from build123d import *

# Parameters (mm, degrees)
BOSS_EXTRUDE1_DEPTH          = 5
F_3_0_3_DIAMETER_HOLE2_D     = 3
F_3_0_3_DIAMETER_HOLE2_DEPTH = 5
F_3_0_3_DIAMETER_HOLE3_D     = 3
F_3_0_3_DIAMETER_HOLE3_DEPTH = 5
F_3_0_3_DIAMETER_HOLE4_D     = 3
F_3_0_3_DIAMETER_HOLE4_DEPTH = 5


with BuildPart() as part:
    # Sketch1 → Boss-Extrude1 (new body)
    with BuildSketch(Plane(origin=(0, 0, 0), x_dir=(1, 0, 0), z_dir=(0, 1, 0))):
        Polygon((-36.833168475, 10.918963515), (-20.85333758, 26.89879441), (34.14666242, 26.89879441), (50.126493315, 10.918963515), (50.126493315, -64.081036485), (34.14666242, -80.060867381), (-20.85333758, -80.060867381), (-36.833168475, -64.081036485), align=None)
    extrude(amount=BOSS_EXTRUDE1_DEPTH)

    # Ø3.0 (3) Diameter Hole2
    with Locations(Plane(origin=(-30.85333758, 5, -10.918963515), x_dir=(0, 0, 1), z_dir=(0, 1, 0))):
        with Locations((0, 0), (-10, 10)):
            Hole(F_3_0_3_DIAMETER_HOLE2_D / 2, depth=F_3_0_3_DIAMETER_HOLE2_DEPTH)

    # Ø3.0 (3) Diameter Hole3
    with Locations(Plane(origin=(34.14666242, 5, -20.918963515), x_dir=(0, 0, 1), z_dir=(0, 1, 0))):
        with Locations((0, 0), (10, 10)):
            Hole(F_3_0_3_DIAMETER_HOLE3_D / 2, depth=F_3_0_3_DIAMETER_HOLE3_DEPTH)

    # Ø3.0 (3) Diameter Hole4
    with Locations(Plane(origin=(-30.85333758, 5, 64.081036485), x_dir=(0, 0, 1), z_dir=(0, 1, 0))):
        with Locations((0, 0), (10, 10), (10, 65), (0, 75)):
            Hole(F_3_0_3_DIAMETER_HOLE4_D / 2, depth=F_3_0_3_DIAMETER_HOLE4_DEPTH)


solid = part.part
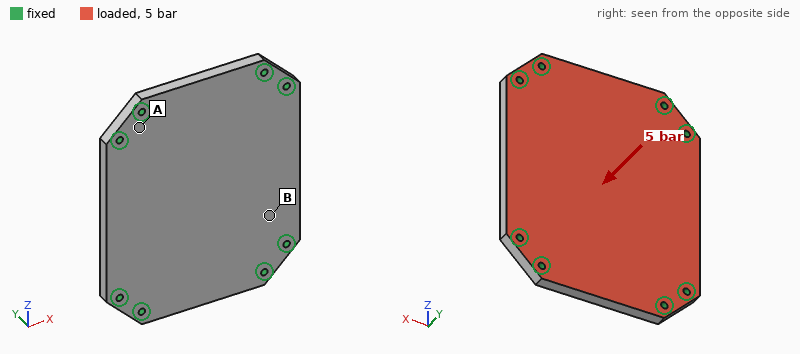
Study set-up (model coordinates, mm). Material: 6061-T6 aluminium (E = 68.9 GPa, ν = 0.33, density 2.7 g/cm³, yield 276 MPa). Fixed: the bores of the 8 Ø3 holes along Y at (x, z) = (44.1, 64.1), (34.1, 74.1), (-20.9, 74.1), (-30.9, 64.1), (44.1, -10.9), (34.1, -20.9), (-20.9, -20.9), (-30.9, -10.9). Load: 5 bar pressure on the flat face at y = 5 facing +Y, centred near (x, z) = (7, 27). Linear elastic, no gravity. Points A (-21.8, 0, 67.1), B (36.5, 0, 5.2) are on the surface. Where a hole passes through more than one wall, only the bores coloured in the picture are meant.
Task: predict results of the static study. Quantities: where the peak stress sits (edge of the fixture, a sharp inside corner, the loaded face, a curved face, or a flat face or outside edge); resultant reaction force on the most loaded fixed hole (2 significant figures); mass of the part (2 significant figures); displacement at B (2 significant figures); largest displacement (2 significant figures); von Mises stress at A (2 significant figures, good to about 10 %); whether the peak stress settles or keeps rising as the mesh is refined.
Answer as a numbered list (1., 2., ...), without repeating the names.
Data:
1. edge of the fixture
2. 700 N
3. 120 g
4. 0.066 mm
5. 0.15 mm
6. 47 MPa
7. keeps rising
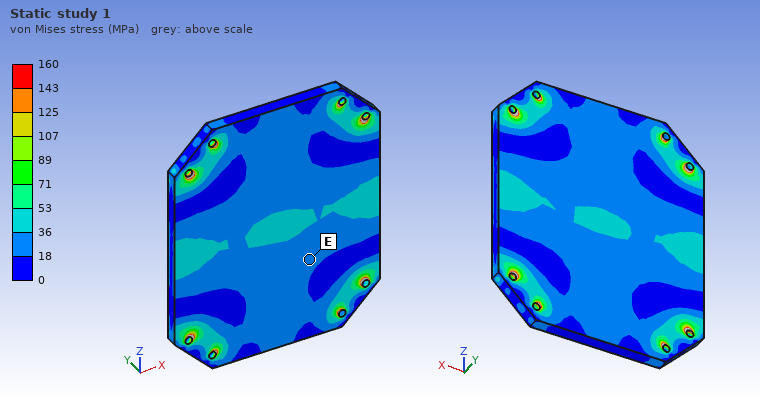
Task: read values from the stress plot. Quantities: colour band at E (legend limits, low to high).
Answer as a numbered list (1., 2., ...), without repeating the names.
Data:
1. 18 to 36 MPa
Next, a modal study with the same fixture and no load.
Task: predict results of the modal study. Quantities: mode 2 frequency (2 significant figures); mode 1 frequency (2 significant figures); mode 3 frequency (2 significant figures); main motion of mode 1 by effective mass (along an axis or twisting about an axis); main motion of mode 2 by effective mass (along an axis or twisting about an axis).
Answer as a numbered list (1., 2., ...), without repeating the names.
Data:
1. 4800 Hz
2. 3100 Hz
3. 6400 Hz
4. along Y
5. twisting about Z
